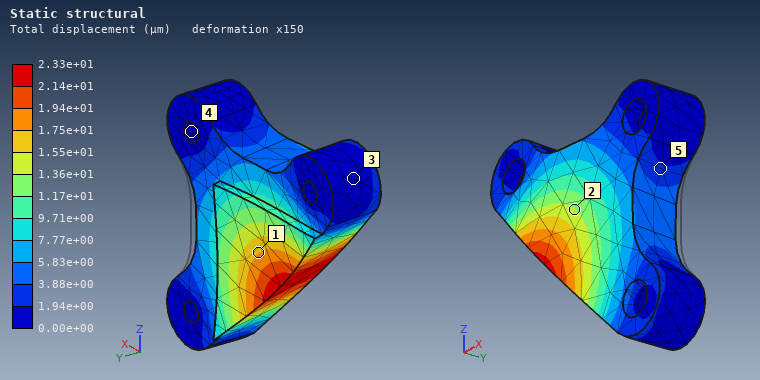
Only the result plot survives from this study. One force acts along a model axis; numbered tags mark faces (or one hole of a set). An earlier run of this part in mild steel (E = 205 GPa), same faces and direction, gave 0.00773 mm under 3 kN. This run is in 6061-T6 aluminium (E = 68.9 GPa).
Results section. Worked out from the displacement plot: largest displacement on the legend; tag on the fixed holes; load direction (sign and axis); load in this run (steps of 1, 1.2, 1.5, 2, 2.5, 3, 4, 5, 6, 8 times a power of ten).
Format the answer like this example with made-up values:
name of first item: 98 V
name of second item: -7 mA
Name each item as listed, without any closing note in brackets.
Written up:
largest displacement on the legend: 2.33e+01 µm
tag on the fixed holes: 4
load direction: -Y
load in this run: 3 kN
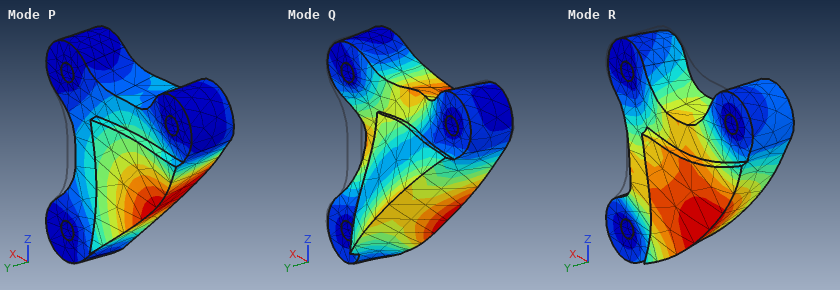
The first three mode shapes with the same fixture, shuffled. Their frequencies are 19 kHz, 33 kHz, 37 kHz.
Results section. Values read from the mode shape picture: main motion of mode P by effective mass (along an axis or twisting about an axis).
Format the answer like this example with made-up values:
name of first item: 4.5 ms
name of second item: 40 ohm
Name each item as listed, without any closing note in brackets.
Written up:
main motion of mode P by effective mass: along Y
